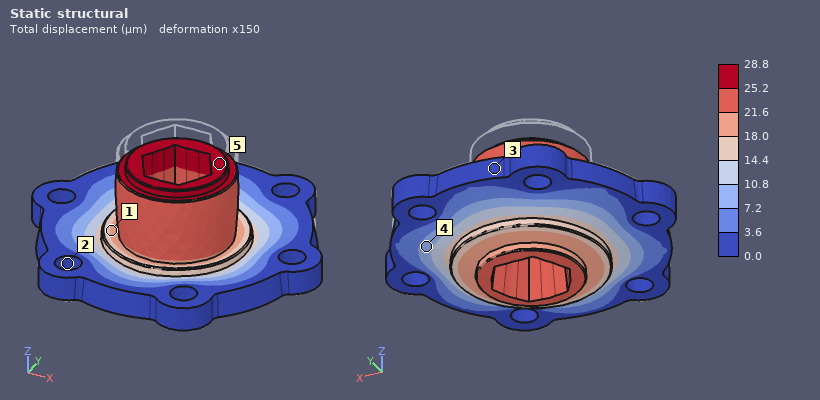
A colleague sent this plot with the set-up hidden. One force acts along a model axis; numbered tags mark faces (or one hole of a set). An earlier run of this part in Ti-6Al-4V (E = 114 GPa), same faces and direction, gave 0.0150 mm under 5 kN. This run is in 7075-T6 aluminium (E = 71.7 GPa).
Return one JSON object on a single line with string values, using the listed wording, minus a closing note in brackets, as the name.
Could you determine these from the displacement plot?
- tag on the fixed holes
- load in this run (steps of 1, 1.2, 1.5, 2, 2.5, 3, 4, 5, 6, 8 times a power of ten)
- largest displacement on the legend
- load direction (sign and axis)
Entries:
{"tag on the fixed holes": "2", "load in this run": "6 kN", "largest displacement on the legend": "28.8 µm", "load direction": "-Z"}
